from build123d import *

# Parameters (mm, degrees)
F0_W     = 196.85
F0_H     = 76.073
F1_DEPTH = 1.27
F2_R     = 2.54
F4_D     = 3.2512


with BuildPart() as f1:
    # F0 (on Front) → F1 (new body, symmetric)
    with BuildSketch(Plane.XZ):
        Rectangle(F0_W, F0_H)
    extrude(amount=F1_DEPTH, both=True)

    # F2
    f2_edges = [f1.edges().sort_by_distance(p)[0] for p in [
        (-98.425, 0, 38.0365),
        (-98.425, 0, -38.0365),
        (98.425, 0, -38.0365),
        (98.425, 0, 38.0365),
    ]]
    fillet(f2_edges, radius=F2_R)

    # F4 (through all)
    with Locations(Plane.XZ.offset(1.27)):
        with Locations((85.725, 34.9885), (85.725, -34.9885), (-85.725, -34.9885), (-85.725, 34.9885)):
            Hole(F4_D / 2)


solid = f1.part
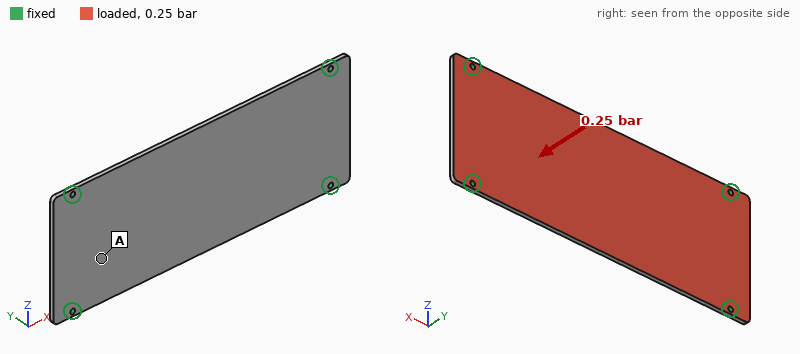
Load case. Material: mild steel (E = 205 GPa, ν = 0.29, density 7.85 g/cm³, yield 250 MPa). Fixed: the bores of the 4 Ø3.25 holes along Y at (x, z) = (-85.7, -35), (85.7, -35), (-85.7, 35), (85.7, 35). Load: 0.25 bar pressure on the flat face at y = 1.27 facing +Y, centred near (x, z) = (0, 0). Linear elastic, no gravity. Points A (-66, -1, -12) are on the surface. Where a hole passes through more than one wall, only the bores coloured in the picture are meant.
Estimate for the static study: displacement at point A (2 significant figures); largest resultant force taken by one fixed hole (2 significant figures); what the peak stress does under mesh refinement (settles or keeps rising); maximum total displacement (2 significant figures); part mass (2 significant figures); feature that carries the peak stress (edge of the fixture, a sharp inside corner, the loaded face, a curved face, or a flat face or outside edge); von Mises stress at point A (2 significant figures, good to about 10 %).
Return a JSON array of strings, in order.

["0.074 mm", "93 N", "keeps rising", "0.28 mm", "300 g", "edge of the fixture", "18 MPa"]
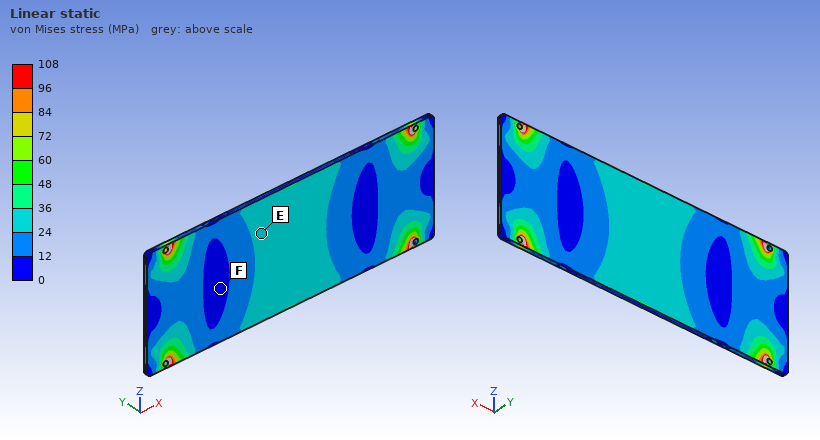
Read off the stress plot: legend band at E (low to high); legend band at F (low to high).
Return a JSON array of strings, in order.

["24 to 36 MPa", "0 to 12 MPa"]
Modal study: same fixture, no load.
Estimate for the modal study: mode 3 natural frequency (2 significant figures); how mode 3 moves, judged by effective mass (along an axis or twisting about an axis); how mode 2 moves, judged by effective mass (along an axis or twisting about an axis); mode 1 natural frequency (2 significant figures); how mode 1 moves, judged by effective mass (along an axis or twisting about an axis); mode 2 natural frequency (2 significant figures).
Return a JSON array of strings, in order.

["1100 Hz", "twisting about Z", "twisting about X", "380 Hz", "along Y", "800 Hz"]
